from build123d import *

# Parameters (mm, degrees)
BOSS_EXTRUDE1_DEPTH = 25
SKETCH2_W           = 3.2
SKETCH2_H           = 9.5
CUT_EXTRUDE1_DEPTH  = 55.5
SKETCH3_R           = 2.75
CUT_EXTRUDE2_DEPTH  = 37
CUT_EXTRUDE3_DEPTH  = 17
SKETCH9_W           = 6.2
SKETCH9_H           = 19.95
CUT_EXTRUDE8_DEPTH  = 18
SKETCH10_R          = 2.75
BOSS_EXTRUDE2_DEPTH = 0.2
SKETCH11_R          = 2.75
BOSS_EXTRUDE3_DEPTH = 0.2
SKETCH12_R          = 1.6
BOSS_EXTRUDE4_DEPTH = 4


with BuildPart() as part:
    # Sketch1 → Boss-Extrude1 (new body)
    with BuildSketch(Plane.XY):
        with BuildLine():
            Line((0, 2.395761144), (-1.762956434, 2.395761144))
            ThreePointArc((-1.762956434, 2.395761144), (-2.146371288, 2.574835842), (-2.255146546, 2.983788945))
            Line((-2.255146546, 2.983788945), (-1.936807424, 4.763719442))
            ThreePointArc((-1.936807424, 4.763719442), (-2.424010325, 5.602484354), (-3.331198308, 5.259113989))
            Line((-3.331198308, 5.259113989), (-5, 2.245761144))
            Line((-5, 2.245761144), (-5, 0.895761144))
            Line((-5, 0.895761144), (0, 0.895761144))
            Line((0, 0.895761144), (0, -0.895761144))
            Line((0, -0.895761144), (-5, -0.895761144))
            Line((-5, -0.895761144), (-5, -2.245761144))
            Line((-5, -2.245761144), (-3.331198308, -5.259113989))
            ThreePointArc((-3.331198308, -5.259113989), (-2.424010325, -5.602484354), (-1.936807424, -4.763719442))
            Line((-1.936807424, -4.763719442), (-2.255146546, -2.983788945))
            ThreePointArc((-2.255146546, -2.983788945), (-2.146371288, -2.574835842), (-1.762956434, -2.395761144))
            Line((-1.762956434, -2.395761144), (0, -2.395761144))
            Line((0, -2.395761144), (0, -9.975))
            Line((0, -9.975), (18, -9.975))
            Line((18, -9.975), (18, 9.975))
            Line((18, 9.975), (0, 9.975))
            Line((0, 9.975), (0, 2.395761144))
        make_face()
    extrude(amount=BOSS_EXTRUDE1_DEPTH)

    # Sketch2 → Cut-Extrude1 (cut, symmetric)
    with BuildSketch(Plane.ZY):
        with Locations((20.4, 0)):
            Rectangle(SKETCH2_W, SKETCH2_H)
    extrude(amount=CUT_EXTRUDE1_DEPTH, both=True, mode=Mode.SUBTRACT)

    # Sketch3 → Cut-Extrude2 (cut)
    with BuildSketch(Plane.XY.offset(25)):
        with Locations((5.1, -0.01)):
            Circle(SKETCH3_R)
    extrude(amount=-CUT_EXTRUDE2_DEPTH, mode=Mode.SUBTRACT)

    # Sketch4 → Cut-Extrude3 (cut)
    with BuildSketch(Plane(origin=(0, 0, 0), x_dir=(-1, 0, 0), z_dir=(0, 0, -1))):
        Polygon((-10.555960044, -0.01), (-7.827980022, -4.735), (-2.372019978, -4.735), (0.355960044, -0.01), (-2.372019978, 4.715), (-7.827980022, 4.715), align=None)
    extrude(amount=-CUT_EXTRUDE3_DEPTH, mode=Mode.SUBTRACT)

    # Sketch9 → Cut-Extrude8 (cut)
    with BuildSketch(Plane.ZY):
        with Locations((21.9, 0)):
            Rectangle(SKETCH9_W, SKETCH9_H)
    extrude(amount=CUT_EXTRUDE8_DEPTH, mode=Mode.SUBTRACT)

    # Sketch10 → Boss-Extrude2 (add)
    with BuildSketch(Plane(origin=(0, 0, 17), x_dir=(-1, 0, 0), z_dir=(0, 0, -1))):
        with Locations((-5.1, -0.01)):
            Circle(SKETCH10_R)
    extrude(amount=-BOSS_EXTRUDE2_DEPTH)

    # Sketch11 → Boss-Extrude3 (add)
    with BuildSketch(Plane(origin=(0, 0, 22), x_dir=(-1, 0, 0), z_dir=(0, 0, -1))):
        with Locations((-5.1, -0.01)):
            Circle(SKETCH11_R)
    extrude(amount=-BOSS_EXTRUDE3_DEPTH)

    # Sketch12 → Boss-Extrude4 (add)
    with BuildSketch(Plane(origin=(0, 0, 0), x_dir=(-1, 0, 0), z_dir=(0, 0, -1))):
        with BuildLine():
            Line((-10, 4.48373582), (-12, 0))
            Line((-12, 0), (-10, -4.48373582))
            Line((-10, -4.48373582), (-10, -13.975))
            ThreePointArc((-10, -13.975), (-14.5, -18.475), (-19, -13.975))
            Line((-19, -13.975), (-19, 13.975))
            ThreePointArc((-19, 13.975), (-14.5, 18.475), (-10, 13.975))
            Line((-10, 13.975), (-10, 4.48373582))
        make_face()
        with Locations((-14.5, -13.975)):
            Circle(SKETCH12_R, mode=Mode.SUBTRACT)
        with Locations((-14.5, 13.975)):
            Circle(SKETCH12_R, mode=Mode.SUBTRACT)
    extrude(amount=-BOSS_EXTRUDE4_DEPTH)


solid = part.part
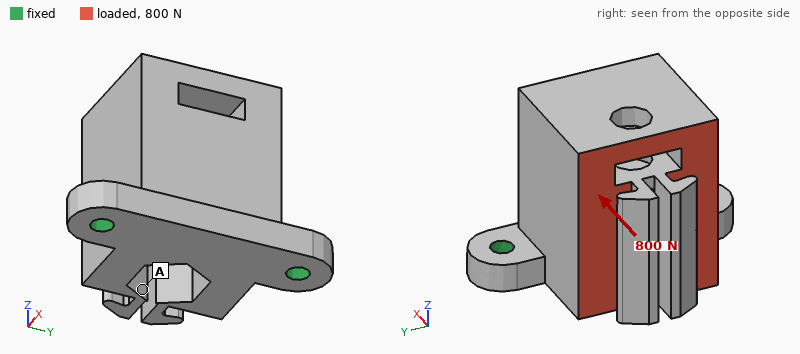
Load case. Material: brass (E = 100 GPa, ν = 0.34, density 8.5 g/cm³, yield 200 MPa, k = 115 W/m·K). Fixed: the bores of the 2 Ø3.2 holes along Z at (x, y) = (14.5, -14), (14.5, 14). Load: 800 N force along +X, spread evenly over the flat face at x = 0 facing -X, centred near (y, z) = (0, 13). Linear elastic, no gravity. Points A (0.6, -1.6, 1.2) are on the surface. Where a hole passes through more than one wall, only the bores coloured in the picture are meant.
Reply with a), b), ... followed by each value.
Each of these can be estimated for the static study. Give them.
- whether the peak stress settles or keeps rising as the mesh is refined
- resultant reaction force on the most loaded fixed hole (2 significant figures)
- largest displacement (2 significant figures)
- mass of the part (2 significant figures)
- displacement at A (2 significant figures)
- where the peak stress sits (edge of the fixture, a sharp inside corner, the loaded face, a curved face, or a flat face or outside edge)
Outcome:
a) keeps rising
b) 400 N
c) 93 µm
d) 69 g
e) 46 µm
f) edge of the fixture
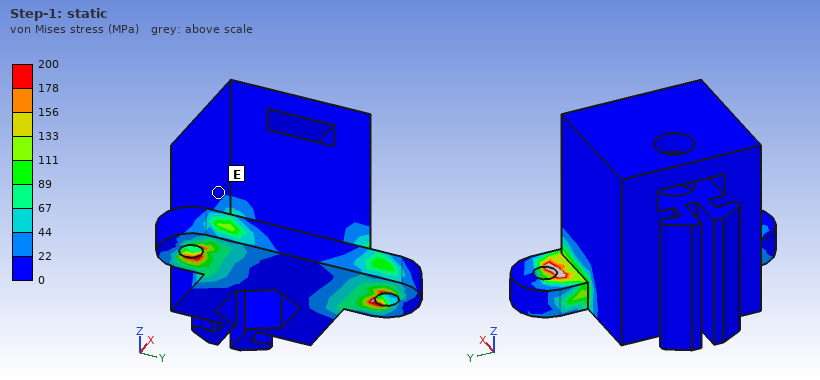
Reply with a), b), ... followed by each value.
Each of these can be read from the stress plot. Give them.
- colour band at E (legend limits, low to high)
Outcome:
a) 0 to 22 MPa
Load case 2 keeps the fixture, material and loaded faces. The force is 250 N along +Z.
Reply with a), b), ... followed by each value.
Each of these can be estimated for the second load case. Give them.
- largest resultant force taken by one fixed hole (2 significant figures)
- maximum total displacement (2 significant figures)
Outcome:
a) 140 N
b) 39 µm
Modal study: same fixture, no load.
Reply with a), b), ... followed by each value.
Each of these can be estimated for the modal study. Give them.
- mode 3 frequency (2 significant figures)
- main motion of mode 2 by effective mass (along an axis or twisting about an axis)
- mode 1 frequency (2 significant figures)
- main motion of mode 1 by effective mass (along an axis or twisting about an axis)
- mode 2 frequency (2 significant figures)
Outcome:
a) 8200 Hz
b) along Y
c) 2100 Hz
d) along X
e) 6800 Hz
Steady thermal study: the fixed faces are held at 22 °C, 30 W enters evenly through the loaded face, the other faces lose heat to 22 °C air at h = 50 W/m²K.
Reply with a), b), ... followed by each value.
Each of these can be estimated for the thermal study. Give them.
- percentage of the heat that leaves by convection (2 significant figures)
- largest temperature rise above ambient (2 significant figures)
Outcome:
a) 17 %
b) 34 K
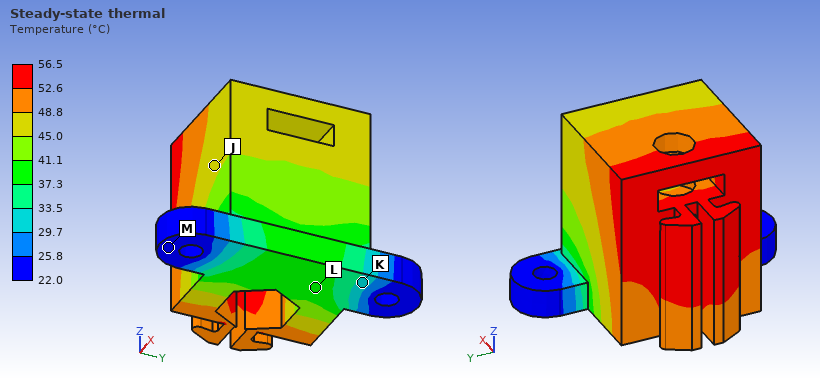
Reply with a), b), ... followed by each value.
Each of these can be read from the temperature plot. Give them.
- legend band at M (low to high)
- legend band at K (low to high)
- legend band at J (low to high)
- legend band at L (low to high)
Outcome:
a) 22.0 to 25.8 °C
b) 29.7 to 33.5 °C
c) 45.0 to 48.8 °C
d) 37.3 to 41.1 °C
